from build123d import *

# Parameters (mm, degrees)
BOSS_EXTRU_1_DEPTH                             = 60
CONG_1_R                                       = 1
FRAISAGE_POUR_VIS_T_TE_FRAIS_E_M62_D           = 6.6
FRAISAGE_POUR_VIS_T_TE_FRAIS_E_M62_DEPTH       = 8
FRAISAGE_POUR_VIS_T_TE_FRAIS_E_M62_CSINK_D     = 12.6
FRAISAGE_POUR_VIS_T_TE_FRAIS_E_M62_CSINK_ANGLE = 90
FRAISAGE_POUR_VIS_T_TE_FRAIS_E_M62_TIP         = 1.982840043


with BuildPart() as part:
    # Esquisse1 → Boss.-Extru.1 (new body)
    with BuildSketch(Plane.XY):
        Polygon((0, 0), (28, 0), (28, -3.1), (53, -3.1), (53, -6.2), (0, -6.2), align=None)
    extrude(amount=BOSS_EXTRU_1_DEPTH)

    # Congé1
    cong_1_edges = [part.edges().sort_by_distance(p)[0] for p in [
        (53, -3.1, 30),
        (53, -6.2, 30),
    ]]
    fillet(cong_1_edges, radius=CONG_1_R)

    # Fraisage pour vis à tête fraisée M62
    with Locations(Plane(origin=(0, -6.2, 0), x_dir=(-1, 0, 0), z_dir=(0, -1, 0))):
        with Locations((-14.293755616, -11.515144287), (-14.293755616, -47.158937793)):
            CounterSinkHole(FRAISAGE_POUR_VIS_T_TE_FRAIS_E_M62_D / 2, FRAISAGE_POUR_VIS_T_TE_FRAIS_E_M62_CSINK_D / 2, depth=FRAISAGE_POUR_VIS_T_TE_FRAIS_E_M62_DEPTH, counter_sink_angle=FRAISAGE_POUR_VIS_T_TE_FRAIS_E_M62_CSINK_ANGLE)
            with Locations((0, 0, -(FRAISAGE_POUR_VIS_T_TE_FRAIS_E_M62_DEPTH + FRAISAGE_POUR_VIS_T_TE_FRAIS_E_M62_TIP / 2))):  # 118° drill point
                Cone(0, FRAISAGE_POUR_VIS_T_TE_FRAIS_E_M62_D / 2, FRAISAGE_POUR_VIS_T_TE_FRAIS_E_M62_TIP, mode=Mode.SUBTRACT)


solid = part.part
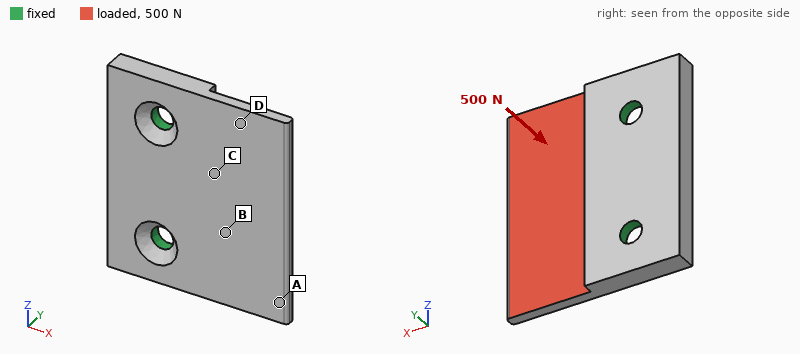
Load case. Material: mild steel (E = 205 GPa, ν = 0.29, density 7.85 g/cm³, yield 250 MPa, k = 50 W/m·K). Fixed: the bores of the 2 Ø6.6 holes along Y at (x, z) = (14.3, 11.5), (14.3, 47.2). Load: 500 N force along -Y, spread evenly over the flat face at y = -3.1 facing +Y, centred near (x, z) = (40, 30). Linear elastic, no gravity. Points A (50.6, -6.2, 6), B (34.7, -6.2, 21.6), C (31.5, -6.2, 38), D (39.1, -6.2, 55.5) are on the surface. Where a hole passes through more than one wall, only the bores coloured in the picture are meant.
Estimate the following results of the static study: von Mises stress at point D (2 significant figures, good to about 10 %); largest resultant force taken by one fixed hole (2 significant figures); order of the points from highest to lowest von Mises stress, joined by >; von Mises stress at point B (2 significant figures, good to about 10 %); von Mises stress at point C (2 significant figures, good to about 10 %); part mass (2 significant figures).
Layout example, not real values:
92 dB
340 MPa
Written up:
18 MPa
270 N
C > B > D > A
30 MPa
40 MPa
110 g
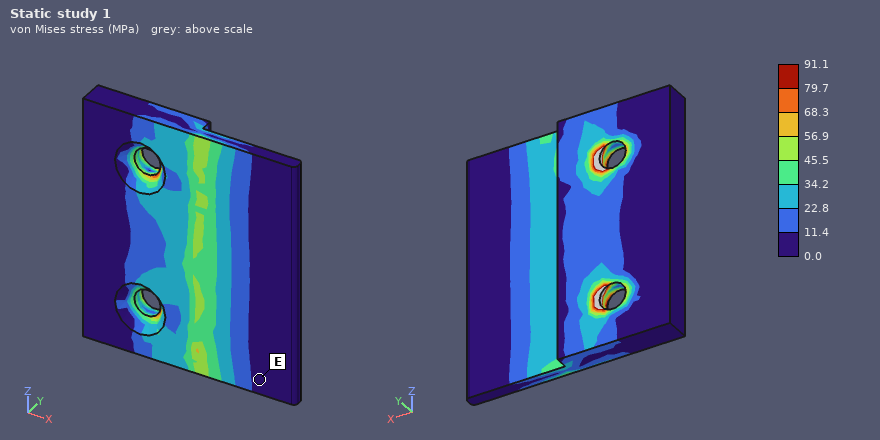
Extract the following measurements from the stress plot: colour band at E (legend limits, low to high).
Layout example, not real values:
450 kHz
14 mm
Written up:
0.0 to 11.4 MPa
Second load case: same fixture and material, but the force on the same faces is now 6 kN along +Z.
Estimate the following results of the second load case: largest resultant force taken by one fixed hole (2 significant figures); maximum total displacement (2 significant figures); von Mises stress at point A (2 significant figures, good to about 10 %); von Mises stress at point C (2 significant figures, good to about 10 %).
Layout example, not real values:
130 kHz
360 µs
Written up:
4.9 kN
60 µm
18 MPa
44 MPa
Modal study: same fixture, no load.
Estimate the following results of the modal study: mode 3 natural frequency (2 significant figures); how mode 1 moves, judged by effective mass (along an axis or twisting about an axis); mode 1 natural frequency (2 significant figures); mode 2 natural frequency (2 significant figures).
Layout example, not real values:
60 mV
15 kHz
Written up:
8200 Hz
along Y
2900 Hz
4400 Hz
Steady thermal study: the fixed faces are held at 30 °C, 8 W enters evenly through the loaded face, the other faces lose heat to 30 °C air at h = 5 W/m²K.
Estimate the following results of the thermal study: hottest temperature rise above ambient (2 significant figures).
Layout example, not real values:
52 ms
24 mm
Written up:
18 K
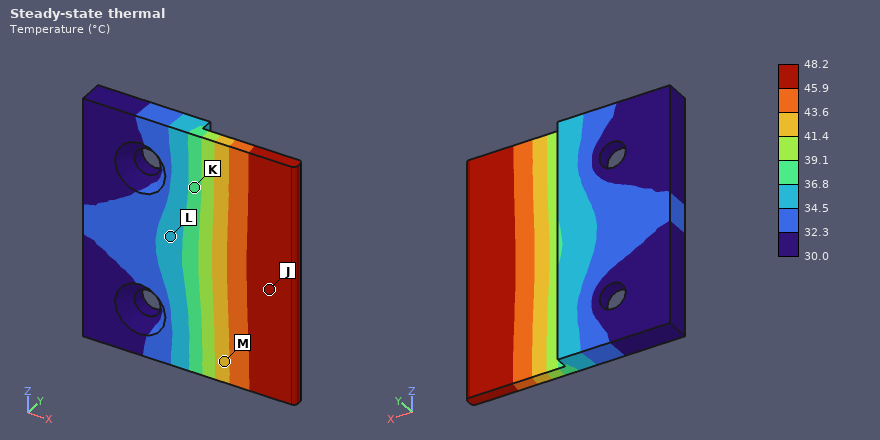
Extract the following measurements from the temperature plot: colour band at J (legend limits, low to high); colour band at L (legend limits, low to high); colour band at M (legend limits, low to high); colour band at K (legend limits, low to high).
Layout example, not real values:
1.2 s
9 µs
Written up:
45.9 to 48.2 °C
34.5 to 36.8 °C
41.4 to 43.6 °C
36.8 to 39.1 °C
